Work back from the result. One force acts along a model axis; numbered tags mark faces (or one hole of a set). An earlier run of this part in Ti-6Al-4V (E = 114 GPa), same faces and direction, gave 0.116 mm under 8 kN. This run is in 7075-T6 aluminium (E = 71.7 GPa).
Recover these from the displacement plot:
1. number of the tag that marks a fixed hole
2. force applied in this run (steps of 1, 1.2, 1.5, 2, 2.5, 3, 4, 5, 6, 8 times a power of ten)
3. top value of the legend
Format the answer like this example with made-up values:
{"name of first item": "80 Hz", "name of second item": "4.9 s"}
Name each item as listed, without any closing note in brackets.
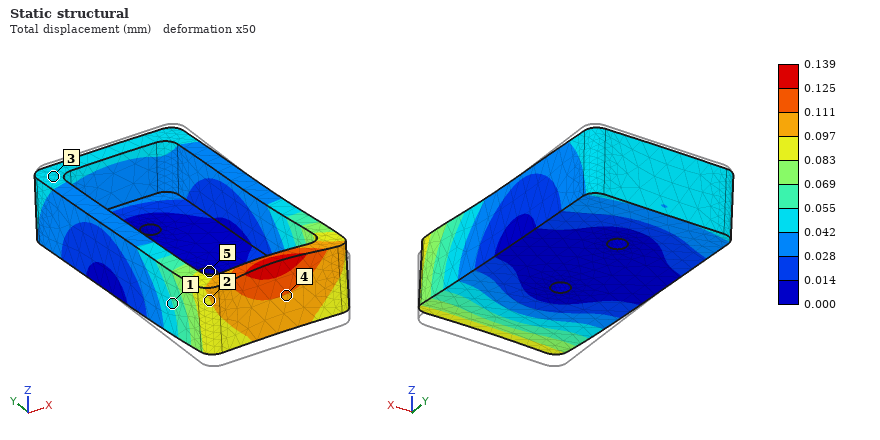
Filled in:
{"number of the tag that marks a fixed hole": "5", "force applied in this run": "6 kN", "top value of the legend": "0.139 mm"}
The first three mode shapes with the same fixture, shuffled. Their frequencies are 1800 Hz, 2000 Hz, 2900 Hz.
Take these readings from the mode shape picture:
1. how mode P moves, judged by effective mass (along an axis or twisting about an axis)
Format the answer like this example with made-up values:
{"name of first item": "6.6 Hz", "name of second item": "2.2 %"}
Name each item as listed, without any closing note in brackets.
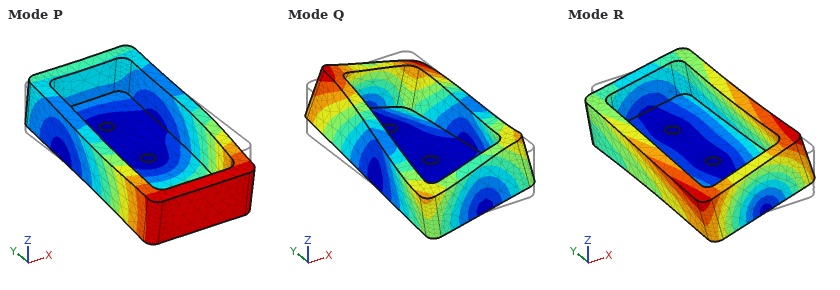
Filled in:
{"how mode P moves, judged by effective mass": "along Z"}
